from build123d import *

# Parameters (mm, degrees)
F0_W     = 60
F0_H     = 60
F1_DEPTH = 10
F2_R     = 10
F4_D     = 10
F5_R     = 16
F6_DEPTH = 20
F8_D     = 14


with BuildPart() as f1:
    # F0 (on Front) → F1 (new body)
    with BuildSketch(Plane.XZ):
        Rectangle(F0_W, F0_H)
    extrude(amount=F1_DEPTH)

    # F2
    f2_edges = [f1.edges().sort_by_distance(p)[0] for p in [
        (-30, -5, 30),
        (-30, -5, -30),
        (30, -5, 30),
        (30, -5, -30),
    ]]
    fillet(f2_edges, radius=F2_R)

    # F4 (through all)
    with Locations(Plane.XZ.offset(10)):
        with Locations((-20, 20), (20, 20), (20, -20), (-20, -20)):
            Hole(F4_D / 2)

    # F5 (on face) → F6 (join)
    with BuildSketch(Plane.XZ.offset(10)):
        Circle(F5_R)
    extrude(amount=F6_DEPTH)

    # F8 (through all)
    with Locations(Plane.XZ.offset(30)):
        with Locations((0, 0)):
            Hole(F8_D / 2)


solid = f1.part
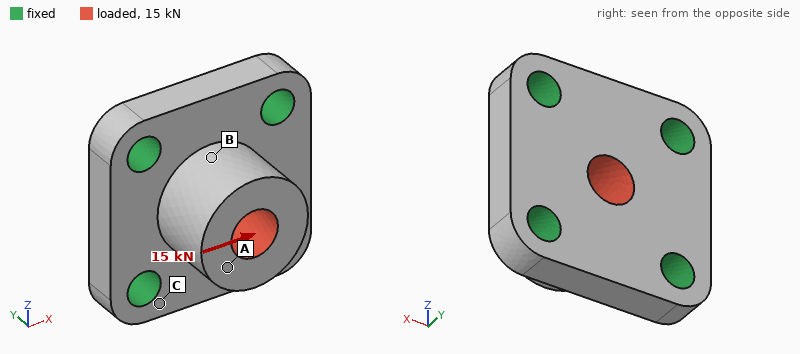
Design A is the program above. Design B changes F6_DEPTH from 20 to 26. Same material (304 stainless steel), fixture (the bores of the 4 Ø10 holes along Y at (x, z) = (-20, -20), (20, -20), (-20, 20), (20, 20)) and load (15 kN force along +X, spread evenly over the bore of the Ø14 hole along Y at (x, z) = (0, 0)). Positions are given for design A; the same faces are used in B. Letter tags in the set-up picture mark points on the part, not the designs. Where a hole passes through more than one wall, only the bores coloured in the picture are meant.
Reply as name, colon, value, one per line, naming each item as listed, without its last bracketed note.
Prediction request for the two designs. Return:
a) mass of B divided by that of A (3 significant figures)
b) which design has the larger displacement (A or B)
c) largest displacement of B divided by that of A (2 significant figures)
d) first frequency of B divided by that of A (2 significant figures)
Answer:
mass of B divided by that of A: 1.09
which design has the larger displacement: B
largest displacement of B divided by that of A: 1.5
first frequency of B divided by that of A: 0.76
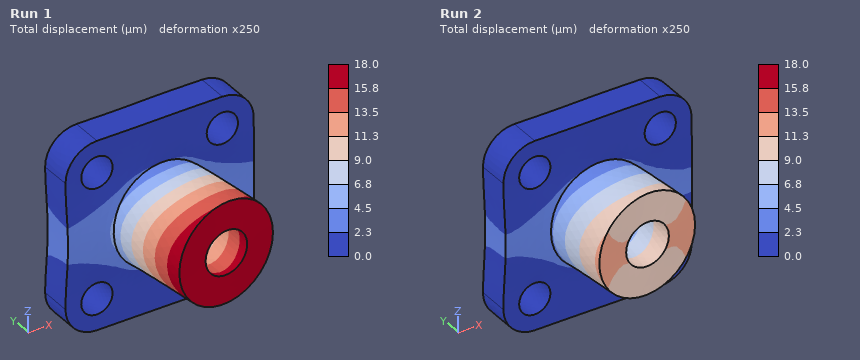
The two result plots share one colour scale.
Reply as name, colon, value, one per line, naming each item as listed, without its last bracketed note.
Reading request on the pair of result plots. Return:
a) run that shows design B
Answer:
run that shows design B: Run 1
